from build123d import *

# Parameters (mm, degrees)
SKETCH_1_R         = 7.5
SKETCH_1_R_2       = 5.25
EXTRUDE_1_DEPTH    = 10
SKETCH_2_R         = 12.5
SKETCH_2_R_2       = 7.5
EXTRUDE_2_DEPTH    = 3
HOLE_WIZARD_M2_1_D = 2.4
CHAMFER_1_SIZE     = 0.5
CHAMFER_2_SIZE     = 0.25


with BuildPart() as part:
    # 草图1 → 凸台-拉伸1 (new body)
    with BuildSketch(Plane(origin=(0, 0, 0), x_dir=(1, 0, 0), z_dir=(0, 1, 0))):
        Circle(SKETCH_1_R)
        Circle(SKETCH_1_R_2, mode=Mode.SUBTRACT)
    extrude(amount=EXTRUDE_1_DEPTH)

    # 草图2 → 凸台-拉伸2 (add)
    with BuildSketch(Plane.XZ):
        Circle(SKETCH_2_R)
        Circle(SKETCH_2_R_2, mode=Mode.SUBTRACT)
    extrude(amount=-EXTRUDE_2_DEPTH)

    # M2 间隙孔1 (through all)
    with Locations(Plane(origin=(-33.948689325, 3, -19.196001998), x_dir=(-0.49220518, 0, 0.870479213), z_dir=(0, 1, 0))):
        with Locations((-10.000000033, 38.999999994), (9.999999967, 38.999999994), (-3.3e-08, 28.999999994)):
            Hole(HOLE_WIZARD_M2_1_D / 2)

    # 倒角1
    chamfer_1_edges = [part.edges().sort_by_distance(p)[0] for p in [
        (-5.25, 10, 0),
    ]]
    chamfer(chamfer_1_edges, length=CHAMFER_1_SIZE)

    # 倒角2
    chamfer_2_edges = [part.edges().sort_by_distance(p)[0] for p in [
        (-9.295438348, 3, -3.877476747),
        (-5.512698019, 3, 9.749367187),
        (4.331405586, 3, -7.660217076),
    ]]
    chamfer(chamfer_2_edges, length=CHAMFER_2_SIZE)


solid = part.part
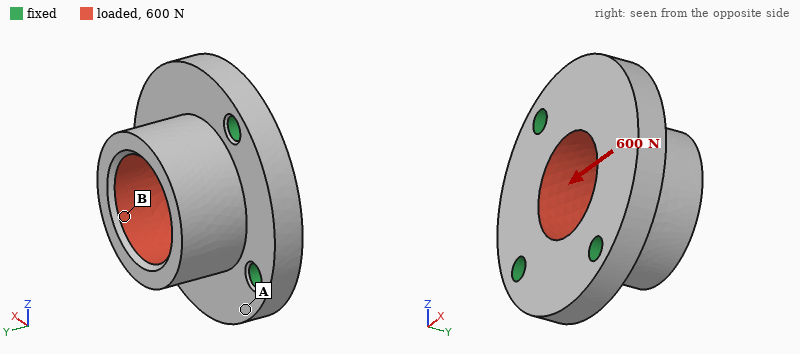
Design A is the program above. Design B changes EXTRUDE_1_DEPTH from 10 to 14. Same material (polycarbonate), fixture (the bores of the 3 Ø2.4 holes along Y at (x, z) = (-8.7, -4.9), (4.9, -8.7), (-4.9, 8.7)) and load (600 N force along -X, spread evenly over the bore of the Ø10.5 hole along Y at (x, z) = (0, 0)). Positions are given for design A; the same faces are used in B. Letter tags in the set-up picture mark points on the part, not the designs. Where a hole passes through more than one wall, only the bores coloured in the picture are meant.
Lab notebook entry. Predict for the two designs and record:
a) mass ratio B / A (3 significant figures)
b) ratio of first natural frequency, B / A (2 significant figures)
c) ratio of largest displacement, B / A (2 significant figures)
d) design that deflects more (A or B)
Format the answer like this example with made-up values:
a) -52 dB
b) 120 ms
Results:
a) 1.20
b) 0.90
c) 1.6
d) B
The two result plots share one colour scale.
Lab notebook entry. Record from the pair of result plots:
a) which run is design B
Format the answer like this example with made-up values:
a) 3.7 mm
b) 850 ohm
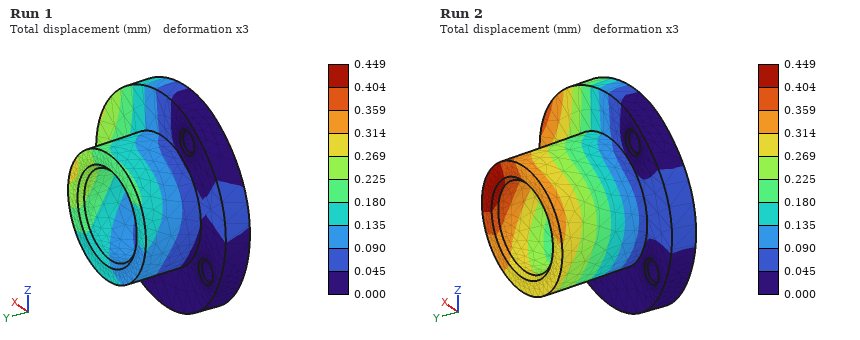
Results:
a) Run 2
